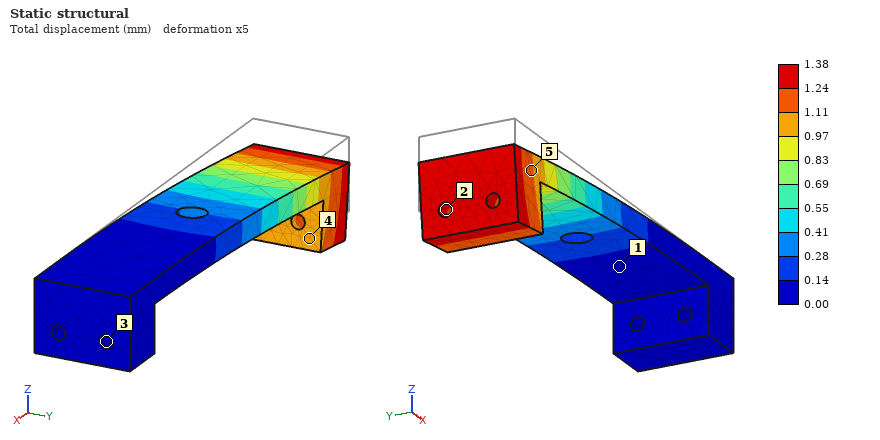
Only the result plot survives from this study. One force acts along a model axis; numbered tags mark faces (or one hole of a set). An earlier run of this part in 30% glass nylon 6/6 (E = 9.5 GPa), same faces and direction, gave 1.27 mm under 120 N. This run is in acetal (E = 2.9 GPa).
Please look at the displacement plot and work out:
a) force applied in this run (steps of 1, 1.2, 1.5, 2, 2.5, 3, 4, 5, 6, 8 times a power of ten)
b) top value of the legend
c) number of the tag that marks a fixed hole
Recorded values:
40 N
1.38 mm
3
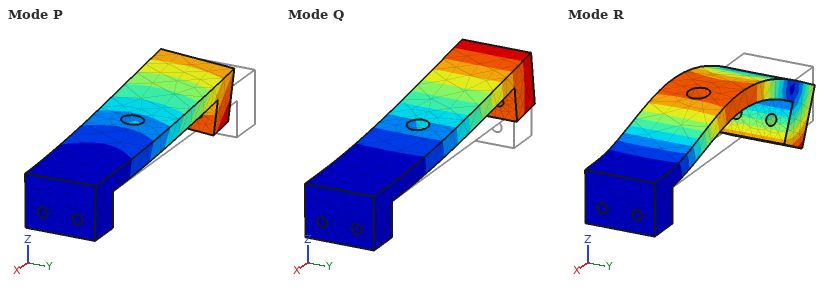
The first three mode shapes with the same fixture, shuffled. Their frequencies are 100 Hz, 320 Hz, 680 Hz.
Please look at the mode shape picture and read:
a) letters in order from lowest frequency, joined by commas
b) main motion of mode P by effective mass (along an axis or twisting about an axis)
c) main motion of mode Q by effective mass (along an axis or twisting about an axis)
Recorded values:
Q, P, R
along Y
along Z
